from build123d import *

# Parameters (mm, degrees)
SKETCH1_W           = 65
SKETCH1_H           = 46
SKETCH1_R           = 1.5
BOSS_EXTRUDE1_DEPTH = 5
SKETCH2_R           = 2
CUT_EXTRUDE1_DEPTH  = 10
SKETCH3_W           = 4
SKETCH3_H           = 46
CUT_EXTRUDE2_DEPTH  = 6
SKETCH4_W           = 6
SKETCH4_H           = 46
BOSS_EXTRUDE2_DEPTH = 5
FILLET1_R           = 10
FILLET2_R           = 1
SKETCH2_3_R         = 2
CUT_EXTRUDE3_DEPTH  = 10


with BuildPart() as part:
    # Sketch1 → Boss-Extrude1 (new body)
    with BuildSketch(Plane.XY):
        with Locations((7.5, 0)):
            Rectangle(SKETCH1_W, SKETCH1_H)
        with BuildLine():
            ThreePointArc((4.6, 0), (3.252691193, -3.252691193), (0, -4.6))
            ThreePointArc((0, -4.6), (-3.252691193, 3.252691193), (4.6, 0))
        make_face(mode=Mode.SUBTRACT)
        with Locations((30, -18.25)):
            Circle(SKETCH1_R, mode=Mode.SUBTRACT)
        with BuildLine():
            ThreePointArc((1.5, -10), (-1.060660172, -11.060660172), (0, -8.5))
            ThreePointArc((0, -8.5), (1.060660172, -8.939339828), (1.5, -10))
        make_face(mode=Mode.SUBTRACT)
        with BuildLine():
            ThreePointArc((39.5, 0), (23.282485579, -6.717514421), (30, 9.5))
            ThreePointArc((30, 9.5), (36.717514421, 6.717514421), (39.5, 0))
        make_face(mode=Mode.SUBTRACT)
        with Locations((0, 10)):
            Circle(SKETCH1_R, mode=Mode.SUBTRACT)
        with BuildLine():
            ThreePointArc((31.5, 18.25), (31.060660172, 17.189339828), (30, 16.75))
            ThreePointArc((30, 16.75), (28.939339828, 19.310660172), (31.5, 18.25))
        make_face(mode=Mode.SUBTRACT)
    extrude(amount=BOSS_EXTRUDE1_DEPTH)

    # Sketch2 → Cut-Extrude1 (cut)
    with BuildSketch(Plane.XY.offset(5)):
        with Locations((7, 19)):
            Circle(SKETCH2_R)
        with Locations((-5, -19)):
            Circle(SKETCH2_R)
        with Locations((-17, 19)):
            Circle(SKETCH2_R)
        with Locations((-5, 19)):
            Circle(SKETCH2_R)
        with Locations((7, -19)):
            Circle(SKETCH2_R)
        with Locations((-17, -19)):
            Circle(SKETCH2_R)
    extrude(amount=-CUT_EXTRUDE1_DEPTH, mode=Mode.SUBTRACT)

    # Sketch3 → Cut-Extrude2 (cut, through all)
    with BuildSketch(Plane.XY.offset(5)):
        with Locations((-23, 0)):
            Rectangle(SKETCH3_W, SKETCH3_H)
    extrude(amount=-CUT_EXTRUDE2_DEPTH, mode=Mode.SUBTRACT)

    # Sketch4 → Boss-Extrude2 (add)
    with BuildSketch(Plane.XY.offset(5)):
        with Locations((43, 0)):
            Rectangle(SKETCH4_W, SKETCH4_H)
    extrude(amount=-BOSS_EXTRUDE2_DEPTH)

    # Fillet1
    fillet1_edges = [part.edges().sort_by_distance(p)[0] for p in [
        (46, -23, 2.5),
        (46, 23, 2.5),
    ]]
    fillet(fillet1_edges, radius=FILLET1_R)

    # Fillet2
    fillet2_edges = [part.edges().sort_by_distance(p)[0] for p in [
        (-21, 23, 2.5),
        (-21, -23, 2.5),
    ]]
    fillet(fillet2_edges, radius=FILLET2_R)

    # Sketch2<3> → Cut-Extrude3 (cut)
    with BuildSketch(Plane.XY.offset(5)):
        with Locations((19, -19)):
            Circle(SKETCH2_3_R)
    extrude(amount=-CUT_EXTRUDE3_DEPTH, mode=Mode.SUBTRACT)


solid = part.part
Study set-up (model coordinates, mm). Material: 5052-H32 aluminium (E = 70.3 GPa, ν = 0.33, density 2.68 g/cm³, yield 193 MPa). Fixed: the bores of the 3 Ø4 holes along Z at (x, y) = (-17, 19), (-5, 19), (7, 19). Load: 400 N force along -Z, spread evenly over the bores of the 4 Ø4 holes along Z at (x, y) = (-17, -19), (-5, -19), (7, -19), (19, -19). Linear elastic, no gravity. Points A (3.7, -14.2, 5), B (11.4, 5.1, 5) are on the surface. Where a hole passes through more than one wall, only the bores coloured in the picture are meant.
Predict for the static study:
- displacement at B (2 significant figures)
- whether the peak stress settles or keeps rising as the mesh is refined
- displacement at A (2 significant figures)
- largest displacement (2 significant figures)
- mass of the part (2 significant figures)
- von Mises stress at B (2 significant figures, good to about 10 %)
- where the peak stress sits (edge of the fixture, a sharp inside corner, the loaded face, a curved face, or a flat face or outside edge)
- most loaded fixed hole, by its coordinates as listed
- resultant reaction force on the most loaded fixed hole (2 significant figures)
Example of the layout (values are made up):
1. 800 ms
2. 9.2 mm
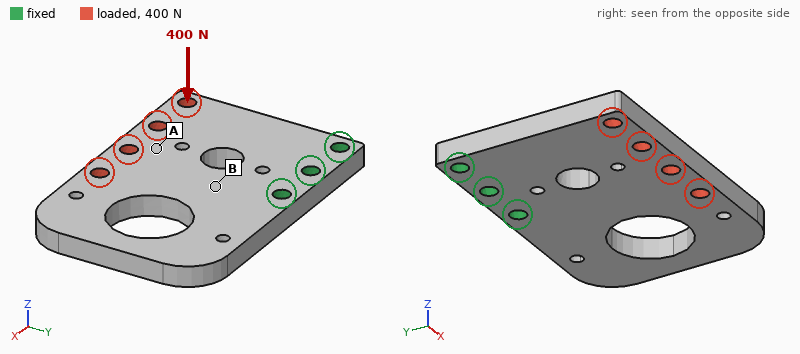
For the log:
1. 0.051 mm
2. keeps rising
3. 0.20 mm
4. 0.28 mm
5. 34 g
6. 49 MPa
7. edge of the fixture
8. (7, 19)
9. 210 N
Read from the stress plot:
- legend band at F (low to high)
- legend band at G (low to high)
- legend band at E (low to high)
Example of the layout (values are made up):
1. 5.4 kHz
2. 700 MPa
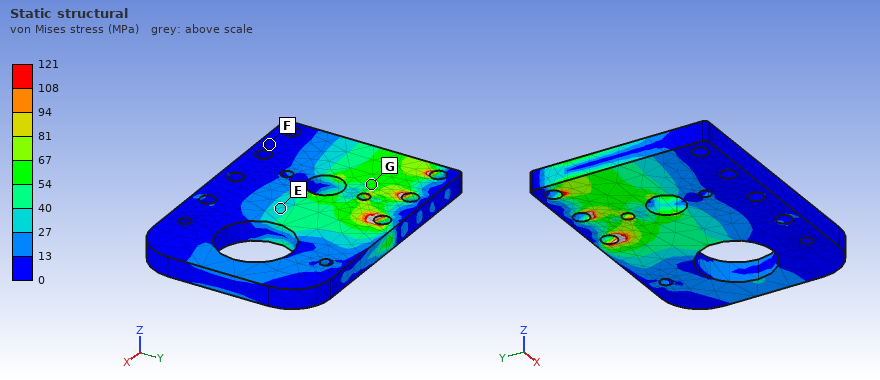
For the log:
1. 0 to 13 MPa
2. 54 to 67 MPa
3. 27 to 40 MPa
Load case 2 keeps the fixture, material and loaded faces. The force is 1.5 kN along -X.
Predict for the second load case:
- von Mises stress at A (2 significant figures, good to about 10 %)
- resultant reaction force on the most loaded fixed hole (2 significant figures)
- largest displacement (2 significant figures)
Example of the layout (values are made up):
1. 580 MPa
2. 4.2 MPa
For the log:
1. 20 MPa
2. 2.1 kN
3. 62 µm
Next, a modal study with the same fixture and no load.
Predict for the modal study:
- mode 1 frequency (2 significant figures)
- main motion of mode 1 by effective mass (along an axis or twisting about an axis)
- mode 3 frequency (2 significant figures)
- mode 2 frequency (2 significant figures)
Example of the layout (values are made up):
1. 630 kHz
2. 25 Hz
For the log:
1. 1600 Hz
2. along Z
3. 4800 Hz
4. 2700 Hz
